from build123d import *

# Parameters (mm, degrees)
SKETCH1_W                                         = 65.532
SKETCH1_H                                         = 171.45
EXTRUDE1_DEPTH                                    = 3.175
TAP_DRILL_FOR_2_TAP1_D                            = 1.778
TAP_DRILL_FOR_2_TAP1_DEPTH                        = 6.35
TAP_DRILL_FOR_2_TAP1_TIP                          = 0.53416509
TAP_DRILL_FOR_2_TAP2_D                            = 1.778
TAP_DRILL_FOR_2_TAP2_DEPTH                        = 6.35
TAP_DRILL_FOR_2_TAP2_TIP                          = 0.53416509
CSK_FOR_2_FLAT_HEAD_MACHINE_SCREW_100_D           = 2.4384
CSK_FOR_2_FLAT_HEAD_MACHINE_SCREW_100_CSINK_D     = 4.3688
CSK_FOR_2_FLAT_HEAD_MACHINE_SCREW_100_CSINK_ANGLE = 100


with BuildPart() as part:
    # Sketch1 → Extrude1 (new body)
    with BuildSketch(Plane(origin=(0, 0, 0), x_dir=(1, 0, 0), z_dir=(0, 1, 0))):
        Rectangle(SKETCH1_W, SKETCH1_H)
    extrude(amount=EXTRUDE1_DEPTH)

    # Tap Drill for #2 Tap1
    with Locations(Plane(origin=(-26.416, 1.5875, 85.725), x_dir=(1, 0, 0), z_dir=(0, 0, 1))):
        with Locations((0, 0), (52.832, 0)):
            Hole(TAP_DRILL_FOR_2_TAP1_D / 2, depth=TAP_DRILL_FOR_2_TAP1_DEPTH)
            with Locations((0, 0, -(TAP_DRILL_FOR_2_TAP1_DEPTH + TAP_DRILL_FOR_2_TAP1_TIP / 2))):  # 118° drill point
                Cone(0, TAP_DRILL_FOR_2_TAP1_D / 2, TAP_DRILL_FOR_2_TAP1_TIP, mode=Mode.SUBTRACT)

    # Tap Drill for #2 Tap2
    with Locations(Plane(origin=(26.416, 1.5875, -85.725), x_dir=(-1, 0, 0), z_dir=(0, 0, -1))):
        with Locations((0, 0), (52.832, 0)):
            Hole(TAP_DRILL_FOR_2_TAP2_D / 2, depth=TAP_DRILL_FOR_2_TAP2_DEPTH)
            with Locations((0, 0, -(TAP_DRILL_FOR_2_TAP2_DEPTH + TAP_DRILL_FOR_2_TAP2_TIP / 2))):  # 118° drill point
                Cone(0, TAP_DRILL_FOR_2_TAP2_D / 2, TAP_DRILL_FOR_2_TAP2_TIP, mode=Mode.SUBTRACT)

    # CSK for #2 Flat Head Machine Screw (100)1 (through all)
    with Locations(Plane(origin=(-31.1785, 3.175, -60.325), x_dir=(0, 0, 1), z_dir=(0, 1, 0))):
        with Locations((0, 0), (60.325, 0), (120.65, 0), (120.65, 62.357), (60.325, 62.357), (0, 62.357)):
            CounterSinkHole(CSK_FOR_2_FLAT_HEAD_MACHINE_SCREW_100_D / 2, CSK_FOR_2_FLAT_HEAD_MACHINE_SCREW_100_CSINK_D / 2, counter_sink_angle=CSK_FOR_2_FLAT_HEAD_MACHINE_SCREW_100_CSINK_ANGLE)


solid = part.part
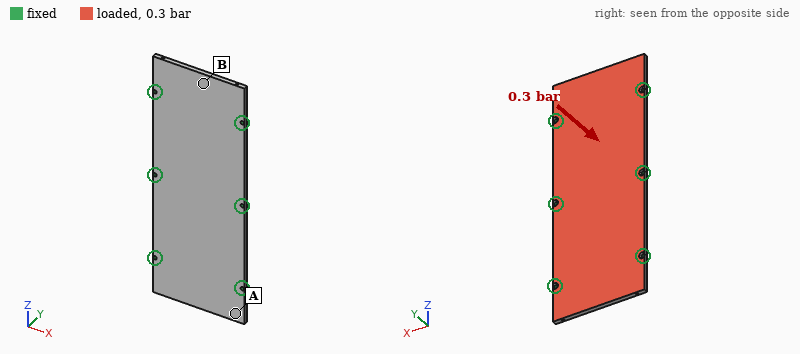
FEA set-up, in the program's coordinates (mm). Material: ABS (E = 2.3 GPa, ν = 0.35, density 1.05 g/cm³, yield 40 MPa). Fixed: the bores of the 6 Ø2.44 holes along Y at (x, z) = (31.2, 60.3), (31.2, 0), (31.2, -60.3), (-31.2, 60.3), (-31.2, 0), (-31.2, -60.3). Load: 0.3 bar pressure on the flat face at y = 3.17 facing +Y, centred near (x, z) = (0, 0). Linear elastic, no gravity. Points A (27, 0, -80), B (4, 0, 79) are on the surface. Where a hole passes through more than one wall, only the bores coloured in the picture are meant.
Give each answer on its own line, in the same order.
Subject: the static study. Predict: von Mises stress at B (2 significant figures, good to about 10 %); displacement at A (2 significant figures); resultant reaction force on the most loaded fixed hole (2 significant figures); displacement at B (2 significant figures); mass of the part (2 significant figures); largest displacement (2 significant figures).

4.5 MPa
0.38 mm
61 N
0.72 mm
37 g
0.84 mm
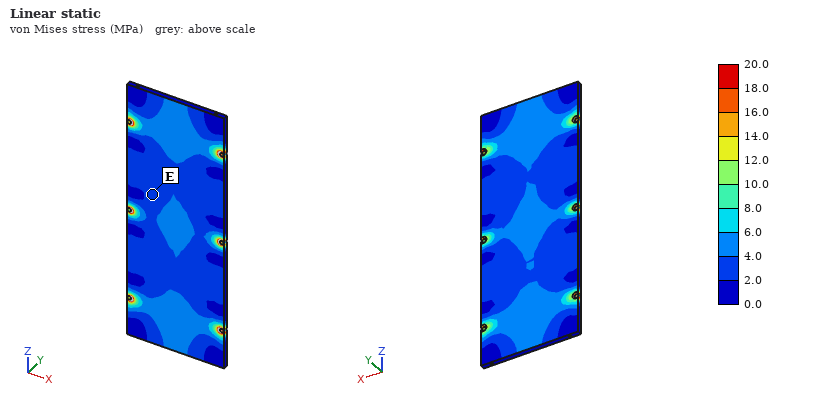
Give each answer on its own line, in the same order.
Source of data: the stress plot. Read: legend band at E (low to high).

2.0 to 4.0 MPa
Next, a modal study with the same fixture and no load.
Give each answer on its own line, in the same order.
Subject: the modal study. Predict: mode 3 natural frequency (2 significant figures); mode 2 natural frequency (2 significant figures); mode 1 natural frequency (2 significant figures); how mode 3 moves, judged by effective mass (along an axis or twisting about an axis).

730 Hz
630 Hz
630 Hz
along Y
